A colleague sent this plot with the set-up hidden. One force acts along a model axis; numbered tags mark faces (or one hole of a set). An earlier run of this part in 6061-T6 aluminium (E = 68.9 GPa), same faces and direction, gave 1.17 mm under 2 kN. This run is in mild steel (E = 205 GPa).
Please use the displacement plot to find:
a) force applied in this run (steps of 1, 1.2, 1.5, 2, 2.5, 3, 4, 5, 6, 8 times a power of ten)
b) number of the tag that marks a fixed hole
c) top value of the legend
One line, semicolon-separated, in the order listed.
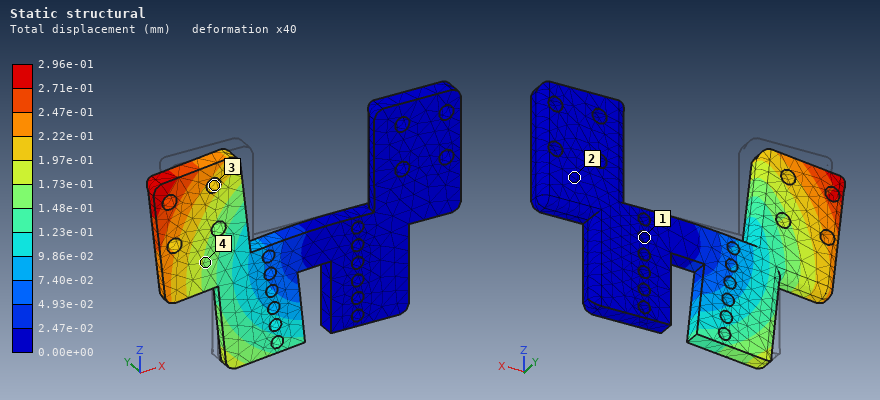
1.5 kN; 1; 2.96e-01 mm
